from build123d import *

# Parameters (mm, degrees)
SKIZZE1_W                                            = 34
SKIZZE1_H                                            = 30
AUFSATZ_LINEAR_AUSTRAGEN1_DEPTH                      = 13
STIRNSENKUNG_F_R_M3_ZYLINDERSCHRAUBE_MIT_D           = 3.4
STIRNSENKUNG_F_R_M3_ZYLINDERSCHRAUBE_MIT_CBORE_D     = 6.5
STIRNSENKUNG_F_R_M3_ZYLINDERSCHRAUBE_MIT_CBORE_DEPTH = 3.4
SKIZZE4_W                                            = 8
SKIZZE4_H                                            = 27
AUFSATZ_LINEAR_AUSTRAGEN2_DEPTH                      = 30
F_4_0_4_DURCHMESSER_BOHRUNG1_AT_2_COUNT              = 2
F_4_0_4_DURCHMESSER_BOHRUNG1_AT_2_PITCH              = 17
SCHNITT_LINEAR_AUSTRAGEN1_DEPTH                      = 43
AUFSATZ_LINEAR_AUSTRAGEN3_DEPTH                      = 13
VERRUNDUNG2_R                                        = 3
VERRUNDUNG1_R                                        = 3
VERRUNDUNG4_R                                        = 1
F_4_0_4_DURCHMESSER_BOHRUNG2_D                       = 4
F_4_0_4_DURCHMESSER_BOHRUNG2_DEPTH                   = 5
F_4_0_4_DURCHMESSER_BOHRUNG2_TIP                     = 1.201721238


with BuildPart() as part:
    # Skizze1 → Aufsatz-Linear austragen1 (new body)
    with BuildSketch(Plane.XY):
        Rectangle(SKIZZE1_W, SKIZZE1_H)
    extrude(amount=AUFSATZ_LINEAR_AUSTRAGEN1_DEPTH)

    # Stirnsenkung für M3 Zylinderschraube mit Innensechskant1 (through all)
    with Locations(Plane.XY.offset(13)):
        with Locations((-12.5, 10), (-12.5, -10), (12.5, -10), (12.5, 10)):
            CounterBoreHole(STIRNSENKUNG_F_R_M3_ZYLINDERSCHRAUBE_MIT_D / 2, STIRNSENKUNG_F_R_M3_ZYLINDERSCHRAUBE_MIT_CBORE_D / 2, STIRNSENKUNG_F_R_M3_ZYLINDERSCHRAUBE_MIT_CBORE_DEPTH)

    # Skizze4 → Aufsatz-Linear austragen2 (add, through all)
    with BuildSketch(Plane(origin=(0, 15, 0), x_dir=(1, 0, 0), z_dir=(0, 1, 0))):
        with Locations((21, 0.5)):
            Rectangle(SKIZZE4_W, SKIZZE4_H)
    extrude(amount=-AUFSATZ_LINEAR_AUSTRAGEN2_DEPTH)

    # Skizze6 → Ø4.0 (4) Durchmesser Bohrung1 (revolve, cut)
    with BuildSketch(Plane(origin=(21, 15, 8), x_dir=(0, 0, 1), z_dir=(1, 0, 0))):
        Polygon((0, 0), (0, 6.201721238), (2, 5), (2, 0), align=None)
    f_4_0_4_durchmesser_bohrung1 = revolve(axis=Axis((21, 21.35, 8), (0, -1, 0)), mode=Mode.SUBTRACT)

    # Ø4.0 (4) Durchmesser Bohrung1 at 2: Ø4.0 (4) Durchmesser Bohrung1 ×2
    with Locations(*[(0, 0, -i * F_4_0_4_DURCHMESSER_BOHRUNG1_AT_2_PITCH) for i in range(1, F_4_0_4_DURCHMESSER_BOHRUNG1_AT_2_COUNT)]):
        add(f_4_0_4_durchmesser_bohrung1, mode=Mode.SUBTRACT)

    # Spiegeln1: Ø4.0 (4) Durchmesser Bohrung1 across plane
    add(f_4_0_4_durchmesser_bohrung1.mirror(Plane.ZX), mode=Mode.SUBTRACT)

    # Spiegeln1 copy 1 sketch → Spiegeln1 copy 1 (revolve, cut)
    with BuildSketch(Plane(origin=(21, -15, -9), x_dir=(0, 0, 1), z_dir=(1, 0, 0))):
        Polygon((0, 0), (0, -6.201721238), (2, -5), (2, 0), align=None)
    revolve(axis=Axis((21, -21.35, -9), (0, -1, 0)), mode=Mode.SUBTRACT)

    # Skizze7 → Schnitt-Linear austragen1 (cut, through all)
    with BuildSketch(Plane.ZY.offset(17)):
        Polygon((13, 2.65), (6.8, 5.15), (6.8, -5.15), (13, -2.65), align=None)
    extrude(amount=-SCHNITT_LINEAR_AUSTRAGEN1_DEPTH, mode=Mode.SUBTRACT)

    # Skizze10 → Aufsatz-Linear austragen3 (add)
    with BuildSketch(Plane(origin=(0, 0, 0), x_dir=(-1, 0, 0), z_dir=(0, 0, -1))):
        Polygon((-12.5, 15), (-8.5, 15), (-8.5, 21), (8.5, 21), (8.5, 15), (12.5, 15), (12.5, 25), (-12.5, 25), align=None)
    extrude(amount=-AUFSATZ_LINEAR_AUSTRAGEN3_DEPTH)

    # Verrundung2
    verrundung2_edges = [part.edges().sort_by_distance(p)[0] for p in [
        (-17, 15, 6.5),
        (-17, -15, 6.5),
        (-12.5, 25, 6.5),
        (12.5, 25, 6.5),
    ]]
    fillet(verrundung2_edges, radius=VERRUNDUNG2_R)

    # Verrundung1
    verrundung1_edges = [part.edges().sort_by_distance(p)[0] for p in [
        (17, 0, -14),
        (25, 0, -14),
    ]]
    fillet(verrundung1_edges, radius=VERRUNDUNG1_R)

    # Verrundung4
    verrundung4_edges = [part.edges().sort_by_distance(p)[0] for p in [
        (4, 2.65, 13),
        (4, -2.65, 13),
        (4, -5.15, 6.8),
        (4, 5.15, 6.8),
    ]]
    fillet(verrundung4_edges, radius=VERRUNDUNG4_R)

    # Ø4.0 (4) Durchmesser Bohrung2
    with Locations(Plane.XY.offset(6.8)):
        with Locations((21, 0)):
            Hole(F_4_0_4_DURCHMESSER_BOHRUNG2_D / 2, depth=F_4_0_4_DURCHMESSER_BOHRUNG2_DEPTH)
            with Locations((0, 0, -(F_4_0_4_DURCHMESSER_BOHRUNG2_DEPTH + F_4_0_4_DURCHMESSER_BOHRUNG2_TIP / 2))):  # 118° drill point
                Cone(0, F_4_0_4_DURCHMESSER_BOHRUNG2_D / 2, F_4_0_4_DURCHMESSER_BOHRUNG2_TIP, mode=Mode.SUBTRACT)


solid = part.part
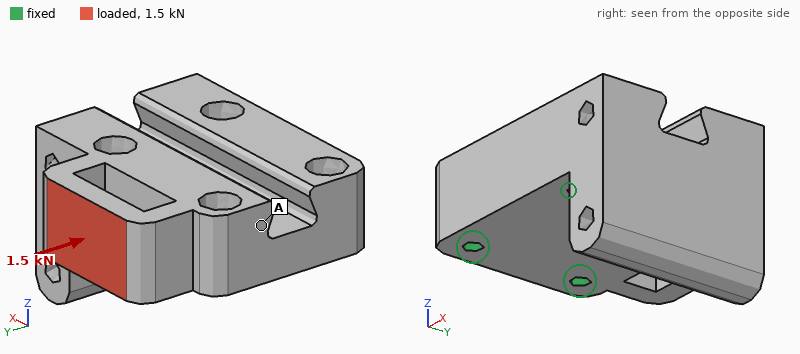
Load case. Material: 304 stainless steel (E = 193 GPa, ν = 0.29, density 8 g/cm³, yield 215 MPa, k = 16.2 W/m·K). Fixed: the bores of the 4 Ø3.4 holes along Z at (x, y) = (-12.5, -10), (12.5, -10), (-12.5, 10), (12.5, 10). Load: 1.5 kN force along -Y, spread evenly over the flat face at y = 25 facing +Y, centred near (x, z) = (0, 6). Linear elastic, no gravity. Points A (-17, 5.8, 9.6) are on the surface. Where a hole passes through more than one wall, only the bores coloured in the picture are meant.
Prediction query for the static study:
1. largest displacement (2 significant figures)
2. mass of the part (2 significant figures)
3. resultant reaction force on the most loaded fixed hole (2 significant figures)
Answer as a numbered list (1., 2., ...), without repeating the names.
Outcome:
1. 6.3 µm
2. 150 g
3. 800 N
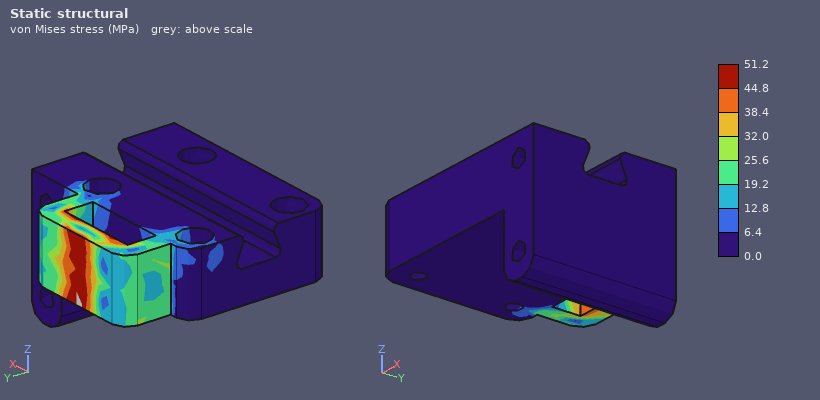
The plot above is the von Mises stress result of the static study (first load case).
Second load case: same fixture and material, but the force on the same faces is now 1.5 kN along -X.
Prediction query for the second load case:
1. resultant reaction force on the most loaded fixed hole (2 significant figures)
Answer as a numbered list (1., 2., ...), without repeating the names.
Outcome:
1. 1.1 kN
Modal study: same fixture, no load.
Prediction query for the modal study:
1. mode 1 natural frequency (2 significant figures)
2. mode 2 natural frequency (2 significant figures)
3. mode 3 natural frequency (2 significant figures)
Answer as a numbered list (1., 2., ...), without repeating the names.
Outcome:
1. 13 kHz
2. 20 kHz
3. 21 kHz
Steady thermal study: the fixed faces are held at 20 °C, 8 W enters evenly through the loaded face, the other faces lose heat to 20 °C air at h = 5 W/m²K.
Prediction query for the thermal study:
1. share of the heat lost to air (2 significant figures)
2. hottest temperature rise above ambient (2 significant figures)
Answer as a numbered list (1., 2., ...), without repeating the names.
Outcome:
1. 3.3 %
2. 72 K
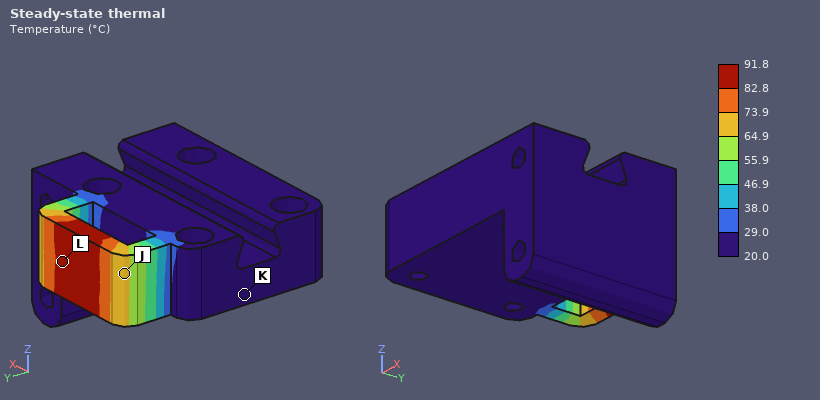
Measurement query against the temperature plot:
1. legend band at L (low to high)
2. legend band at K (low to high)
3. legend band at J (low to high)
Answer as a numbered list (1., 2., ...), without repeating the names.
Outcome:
1. 82.8 to 91.8 °C
2. 20.0 to 29.0 °C
3. 64.9 to 73.9 °C
